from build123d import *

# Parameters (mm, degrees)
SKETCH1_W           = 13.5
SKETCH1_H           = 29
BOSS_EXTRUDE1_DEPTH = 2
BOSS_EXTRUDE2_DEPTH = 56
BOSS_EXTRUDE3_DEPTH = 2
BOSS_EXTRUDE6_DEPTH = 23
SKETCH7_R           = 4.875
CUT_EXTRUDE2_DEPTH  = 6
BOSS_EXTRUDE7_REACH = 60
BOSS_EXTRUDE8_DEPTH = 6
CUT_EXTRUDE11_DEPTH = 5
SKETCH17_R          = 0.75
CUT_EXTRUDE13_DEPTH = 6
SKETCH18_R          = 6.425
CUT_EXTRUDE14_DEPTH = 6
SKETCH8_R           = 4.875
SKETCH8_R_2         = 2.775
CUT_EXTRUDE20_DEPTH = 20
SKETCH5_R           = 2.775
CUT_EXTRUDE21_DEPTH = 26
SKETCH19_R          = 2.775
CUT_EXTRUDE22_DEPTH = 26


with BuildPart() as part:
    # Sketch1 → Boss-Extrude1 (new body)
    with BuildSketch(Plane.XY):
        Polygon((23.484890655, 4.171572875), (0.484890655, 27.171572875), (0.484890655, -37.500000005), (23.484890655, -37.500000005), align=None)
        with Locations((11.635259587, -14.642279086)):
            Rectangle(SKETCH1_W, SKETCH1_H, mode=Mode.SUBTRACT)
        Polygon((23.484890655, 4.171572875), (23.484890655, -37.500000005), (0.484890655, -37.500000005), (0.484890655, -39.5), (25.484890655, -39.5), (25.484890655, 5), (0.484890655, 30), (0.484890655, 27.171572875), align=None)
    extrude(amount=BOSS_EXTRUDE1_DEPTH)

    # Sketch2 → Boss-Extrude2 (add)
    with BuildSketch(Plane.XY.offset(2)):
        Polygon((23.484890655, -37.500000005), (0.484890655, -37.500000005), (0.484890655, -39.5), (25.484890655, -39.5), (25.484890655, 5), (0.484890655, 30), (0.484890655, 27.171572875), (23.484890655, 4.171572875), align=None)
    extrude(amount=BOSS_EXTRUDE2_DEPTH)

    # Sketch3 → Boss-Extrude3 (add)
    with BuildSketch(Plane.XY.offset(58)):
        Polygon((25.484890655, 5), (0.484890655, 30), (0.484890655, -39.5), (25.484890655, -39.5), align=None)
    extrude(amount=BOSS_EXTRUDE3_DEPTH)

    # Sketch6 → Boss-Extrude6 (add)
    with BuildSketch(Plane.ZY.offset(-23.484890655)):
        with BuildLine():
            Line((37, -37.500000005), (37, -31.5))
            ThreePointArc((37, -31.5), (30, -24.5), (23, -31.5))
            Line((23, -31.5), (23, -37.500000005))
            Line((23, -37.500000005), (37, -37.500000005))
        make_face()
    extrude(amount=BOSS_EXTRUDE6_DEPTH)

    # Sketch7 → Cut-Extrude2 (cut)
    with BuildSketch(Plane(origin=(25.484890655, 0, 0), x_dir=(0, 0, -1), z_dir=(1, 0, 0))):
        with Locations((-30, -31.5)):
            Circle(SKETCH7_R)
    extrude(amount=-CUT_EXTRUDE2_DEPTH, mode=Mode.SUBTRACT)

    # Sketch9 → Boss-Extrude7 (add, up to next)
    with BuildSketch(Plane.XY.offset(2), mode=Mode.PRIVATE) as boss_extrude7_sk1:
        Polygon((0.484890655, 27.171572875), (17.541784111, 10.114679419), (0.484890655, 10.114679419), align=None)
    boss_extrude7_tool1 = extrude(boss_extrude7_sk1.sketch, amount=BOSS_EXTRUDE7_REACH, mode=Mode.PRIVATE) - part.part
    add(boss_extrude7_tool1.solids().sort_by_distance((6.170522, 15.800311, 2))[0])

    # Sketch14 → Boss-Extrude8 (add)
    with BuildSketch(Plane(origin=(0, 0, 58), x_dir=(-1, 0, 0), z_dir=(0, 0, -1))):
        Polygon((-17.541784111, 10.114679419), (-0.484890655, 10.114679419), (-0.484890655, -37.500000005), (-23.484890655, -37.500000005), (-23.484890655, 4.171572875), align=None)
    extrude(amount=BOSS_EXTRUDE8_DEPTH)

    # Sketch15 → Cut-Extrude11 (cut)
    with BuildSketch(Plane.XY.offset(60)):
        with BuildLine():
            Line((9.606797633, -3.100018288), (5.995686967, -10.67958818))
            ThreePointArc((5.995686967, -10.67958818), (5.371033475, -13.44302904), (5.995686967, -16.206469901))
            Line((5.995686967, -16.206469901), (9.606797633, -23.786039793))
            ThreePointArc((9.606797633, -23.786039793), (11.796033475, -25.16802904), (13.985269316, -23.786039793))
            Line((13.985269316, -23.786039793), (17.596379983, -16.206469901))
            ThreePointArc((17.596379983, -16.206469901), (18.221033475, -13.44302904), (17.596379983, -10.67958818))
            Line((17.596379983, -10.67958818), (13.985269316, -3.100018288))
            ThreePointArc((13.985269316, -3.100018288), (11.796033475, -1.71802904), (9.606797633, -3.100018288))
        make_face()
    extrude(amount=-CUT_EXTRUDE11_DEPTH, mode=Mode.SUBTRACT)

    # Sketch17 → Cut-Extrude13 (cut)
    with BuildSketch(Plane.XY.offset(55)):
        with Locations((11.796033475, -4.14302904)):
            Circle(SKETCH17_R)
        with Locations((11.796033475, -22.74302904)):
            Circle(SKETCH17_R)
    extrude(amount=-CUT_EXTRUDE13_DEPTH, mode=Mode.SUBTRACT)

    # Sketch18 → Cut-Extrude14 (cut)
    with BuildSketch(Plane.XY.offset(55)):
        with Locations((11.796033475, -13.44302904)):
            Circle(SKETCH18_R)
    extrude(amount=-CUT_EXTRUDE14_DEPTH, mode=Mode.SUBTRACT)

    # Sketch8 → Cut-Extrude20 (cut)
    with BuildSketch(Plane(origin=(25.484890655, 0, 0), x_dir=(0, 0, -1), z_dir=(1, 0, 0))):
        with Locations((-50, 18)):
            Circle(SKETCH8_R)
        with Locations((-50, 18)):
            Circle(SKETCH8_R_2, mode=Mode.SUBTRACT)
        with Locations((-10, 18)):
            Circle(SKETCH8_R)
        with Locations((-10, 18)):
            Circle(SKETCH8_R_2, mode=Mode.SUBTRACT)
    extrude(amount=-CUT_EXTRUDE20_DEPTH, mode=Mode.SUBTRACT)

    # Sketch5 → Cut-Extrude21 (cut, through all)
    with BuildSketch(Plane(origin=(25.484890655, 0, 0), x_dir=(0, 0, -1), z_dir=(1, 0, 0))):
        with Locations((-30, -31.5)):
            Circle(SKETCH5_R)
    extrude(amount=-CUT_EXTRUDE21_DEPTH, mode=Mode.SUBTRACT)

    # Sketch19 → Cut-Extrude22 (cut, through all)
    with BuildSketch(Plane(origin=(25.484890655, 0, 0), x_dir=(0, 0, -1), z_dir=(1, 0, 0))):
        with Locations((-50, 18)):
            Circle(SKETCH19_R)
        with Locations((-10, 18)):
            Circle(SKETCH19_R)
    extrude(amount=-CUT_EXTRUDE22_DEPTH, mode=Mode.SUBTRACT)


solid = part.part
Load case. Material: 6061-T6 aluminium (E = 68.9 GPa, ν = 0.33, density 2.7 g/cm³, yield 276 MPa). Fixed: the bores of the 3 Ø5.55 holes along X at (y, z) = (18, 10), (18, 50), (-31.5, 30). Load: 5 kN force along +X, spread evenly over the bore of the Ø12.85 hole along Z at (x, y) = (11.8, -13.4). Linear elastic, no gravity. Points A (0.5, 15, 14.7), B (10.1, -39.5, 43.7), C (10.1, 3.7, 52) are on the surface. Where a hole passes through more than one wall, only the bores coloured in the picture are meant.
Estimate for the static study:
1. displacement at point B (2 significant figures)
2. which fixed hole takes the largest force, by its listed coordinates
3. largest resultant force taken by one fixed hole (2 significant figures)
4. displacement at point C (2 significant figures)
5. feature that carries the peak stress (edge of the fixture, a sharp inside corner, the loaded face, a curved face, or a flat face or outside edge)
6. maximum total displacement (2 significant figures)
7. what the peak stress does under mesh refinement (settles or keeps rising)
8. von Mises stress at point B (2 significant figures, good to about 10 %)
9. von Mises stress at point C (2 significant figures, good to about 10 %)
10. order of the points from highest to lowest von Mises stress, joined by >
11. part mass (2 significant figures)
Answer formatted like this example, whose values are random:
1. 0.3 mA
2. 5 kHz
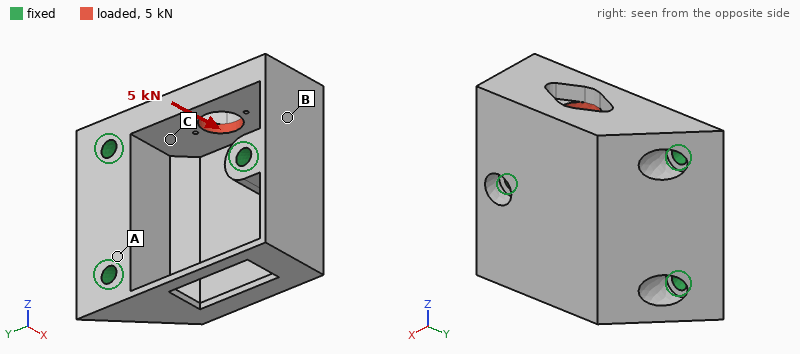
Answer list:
1. 33 µm
2. (18, 50)
3. 3.8 kN
4. 39 µm
5. edge of the fixture
6. 85 µm
7. keeps rising
8. 97 MPa
9. 45 MPa
10. B > C > A
11. 84 g
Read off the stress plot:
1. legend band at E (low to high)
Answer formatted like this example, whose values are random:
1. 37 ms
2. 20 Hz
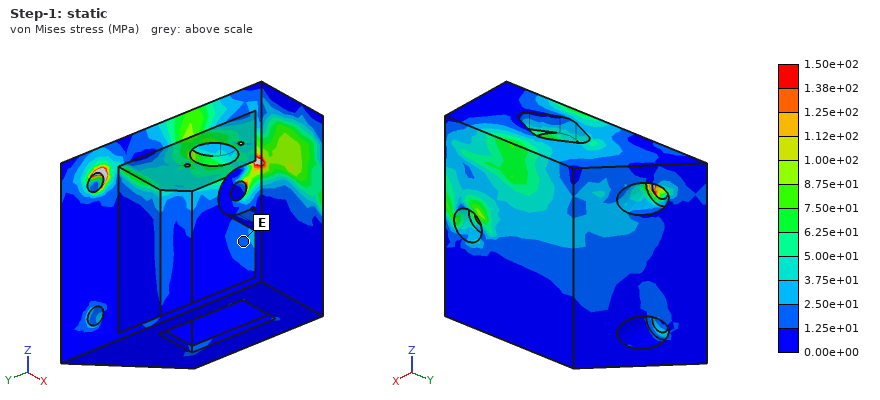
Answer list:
1. 1.25e+01 to 2.50e+01 MPa
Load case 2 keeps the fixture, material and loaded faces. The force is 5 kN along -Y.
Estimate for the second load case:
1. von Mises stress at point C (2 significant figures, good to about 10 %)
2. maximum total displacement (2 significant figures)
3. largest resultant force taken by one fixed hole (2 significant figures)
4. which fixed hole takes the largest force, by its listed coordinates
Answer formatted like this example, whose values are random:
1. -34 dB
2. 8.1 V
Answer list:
1. 38 MPa
2. 38 µm
3. 3.8 kN
4. (18, 50)
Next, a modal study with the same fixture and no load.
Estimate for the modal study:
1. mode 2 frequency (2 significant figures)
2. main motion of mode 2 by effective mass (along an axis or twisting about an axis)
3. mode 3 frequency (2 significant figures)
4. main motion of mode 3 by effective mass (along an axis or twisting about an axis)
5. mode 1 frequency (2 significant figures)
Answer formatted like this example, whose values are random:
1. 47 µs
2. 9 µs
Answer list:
1. 7700 Hz
2. along X
3. 8700 Hz
4. along X
5. 5300 Hz
